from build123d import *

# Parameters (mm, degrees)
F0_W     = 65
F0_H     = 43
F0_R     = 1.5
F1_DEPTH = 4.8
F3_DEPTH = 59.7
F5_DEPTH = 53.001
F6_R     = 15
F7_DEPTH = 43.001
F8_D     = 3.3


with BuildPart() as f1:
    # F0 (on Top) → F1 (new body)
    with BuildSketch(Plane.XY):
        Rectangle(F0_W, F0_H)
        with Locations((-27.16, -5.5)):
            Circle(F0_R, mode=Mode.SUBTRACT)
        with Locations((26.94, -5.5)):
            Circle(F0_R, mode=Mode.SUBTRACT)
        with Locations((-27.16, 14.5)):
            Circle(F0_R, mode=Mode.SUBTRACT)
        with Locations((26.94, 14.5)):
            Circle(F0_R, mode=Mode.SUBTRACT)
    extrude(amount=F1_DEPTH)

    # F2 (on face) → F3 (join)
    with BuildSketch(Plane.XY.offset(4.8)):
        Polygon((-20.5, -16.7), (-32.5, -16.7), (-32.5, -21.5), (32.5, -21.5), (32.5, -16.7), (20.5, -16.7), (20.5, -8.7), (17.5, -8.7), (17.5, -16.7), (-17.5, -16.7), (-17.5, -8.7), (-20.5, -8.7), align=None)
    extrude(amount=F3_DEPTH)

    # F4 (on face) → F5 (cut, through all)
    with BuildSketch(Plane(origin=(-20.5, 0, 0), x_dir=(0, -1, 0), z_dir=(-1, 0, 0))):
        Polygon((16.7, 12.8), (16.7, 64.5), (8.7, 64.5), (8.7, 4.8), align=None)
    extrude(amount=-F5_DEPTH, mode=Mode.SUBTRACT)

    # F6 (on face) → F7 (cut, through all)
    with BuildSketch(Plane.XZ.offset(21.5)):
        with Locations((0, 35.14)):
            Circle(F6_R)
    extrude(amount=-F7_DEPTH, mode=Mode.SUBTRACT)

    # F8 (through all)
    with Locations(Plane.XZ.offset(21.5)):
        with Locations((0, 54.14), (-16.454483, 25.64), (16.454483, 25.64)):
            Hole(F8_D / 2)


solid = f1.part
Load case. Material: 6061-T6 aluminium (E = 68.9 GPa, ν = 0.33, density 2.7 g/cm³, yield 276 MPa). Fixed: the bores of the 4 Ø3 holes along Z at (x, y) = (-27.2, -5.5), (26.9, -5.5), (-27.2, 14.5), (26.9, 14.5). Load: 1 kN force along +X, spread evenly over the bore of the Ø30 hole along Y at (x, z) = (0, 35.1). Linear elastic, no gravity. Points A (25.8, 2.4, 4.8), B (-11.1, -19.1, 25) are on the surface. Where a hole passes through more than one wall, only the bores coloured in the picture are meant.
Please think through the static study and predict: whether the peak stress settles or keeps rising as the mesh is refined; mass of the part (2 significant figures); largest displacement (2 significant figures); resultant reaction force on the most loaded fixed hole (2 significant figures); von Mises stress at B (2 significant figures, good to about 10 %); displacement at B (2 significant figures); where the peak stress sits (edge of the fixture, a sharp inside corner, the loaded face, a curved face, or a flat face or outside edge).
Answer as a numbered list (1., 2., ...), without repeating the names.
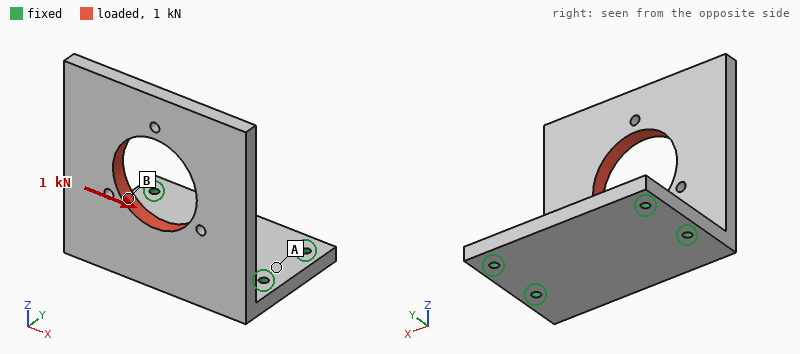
1. keeps rising
2. 77 g
3. 0.12 mm
4. 830 N
5. 22 MPa
6. 0.037 mm
7. edge of the fixture
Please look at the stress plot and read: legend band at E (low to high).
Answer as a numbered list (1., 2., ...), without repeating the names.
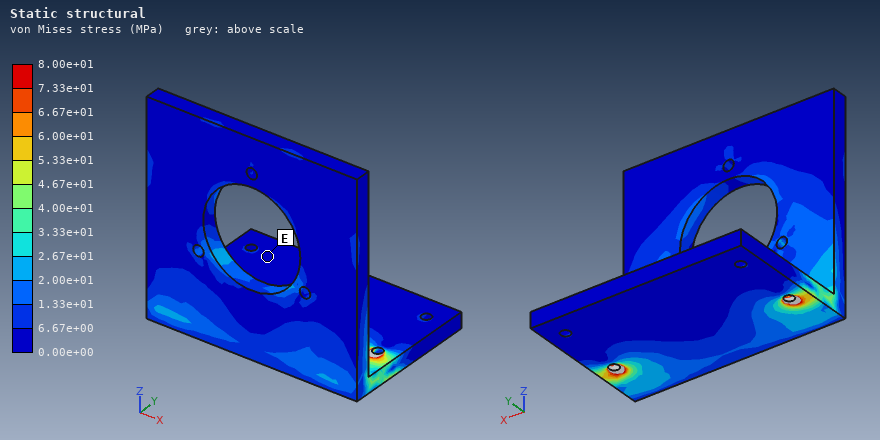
1. 0.00e+00 to 6.67e+00 MPa
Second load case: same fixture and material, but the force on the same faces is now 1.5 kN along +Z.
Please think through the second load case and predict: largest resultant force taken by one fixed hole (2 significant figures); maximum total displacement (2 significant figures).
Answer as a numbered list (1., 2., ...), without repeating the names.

1. 960 N
2. 0.28 mm
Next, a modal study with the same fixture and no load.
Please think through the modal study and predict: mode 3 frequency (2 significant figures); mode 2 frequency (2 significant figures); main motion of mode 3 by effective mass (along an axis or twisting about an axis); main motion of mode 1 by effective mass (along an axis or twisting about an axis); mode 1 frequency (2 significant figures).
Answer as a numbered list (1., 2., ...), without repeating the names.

1. 3100 Hz
2. 1900 Hz
3. along X
4. along Y
5. 800 Hz
